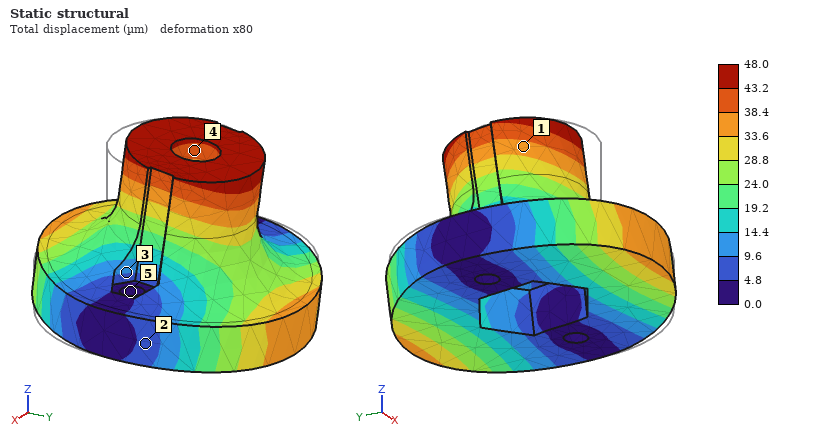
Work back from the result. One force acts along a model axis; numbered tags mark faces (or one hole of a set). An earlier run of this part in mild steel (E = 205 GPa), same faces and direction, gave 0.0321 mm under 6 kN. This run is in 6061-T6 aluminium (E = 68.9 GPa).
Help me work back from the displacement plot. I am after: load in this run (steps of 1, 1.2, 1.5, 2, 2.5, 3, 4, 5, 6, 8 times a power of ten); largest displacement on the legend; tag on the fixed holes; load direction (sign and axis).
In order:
3 kN
48.0 µm
5
+Y
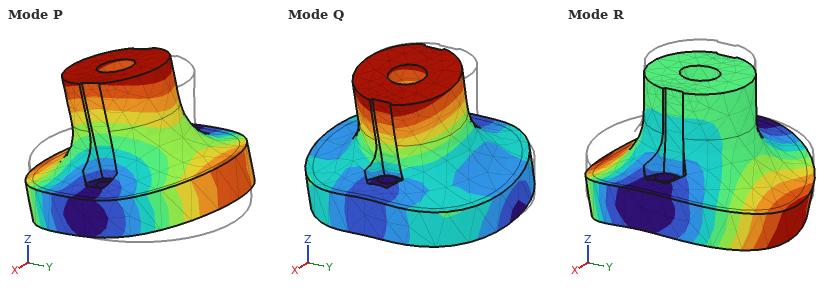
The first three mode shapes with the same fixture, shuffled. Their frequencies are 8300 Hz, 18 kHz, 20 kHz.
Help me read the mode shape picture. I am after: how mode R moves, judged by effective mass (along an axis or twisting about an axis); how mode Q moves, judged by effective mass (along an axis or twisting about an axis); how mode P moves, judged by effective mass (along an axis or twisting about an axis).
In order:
along Z
along X
along Y
